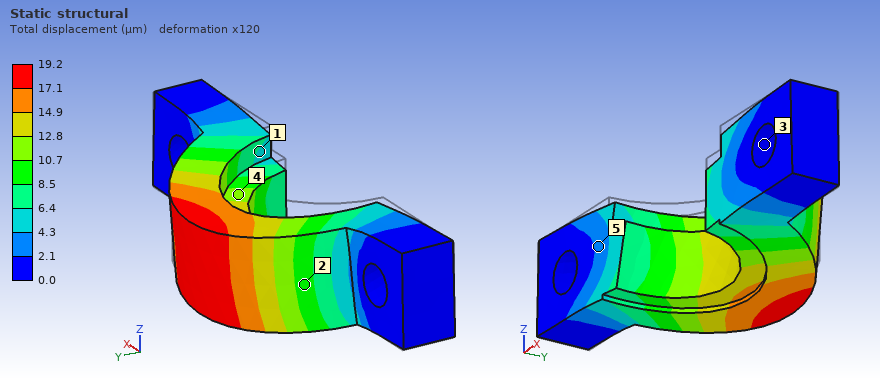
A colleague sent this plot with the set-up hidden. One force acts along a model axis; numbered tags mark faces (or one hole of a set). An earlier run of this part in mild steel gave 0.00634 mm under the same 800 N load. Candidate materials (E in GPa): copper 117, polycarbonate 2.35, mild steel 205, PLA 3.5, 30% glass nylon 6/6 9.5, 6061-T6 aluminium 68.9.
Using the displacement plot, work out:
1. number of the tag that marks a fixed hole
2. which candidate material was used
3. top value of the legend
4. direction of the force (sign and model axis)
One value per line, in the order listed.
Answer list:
3
6061-T6 aluminium
19.2 µm
-Z
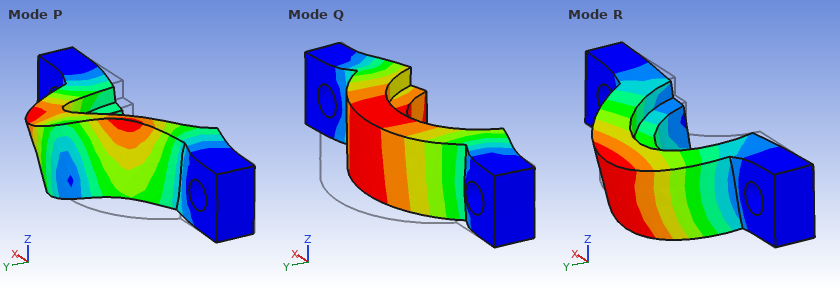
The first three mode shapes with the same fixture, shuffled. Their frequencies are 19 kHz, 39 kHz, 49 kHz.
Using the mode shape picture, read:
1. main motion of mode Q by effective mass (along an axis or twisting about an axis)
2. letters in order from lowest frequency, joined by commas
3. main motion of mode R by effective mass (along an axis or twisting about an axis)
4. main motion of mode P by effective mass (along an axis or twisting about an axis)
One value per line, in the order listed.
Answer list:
along Y
R, Q, P
along Z
along X
